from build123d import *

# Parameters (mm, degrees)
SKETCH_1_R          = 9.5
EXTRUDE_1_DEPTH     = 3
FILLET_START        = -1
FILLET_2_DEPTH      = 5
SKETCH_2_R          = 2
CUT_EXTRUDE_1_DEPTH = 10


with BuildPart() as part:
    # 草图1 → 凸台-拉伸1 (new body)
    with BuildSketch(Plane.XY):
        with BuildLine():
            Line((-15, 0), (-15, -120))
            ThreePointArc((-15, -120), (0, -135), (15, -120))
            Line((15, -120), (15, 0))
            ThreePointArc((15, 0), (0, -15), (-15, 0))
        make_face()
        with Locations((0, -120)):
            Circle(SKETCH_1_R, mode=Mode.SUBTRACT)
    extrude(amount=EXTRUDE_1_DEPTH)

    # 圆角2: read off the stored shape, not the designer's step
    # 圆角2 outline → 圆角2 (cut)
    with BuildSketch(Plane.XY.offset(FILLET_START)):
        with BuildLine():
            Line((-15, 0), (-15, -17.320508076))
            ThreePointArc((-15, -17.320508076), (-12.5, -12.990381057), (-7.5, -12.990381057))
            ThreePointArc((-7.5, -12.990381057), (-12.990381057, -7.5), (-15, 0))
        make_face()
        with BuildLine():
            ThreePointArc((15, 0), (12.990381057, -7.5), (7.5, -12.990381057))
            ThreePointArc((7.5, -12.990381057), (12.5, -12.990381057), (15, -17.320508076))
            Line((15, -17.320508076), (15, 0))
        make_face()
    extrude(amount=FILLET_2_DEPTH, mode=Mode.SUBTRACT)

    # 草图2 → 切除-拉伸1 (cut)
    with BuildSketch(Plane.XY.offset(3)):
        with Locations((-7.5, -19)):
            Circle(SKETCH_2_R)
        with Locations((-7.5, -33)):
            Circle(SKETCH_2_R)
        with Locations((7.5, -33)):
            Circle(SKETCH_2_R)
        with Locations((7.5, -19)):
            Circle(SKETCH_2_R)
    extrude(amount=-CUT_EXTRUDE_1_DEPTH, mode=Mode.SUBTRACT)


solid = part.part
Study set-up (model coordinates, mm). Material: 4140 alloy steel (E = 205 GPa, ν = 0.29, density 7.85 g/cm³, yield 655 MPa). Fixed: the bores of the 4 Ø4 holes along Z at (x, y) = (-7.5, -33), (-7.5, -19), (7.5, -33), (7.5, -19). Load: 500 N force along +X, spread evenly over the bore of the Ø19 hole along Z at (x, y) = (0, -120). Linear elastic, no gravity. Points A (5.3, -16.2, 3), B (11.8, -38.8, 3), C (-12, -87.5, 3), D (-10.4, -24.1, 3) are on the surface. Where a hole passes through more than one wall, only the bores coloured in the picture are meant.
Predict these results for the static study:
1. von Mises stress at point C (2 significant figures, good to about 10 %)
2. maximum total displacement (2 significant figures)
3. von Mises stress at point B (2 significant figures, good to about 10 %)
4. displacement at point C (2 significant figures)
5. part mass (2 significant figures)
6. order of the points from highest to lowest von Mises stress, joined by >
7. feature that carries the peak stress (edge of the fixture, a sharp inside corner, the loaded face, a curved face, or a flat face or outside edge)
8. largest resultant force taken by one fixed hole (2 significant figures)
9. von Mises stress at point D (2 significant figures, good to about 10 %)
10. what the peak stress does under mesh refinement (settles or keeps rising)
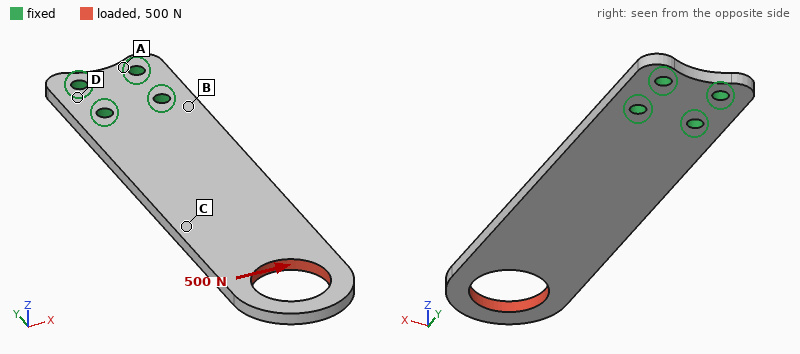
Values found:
29 MPa
0.12 mm
67 MPa
0.048 mm
76 g
B > C > D > A
edge of the fixture
2.0 kN
20 MPa
keeps rising
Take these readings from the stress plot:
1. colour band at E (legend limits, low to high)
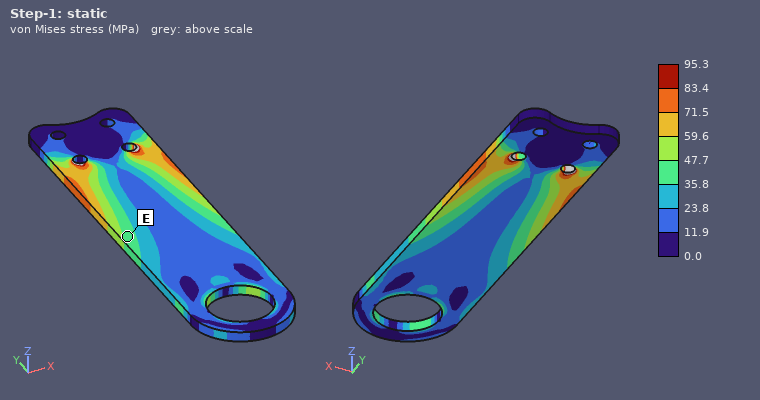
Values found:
35.8 to 47.7 MPa
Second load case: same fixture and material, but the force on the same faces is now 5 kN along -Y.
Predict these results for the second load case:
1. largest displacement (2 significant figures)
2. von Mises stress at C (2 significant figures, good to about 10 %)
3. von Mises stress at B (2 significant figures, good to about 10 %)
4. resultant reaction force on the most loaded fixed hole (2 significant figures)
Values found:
43 µm
59 MPa
51 MPa
2.2 kN
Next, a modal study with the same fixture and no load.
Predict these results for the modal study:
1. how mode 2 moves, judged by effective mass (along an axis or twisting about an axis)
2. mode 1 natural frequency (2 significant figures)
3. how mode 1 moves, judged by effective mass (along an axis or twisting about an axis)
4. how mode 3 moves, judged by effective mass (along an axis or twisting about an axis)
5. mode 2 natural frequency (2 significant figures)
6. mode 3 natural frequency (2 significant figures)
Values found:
along Z
300 Hz
along Z
twisting about Y
1700 Hz
1800 Hz
